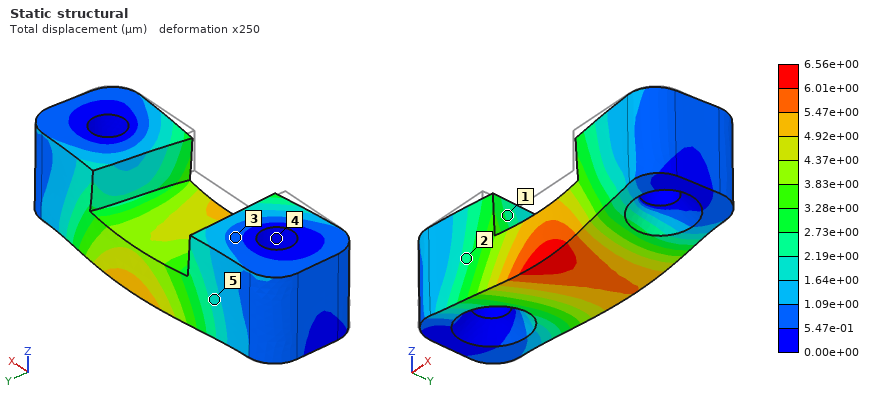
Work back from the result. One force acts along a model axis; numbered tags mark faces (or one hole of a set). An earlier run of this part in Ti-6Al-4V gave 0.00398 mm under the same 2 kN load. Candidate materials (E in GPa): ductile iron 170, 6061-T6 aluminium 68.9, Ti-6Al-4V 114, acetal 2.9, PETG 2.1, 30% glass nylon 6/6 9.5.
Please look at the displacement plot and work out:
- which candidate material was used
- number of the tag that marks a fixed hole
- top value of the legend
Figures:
6061-T6 aluminium
4
6.56e+00 µm
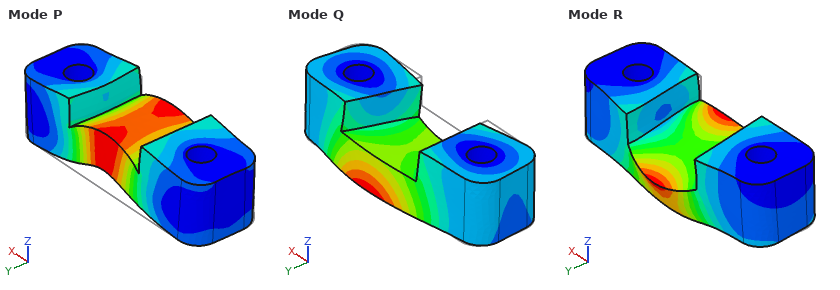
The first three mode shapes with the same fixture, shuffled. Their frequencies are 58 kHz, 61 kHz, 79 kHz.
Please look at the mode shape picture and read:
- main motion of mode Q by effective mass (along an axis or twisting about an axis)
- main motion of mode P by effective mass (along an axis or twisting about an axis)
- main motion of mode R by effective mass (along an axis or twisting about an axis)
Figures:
along Y
along Z
twisting about X
